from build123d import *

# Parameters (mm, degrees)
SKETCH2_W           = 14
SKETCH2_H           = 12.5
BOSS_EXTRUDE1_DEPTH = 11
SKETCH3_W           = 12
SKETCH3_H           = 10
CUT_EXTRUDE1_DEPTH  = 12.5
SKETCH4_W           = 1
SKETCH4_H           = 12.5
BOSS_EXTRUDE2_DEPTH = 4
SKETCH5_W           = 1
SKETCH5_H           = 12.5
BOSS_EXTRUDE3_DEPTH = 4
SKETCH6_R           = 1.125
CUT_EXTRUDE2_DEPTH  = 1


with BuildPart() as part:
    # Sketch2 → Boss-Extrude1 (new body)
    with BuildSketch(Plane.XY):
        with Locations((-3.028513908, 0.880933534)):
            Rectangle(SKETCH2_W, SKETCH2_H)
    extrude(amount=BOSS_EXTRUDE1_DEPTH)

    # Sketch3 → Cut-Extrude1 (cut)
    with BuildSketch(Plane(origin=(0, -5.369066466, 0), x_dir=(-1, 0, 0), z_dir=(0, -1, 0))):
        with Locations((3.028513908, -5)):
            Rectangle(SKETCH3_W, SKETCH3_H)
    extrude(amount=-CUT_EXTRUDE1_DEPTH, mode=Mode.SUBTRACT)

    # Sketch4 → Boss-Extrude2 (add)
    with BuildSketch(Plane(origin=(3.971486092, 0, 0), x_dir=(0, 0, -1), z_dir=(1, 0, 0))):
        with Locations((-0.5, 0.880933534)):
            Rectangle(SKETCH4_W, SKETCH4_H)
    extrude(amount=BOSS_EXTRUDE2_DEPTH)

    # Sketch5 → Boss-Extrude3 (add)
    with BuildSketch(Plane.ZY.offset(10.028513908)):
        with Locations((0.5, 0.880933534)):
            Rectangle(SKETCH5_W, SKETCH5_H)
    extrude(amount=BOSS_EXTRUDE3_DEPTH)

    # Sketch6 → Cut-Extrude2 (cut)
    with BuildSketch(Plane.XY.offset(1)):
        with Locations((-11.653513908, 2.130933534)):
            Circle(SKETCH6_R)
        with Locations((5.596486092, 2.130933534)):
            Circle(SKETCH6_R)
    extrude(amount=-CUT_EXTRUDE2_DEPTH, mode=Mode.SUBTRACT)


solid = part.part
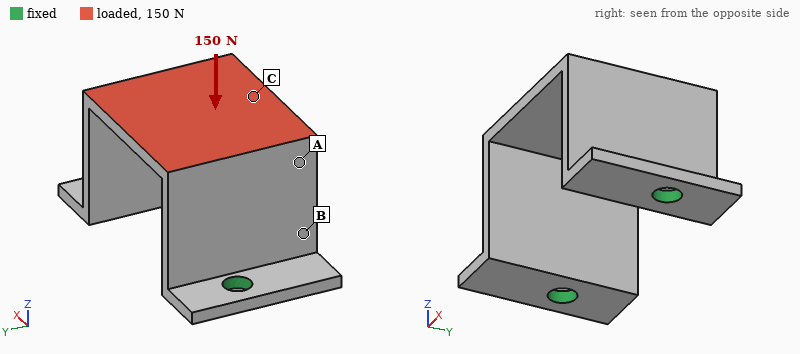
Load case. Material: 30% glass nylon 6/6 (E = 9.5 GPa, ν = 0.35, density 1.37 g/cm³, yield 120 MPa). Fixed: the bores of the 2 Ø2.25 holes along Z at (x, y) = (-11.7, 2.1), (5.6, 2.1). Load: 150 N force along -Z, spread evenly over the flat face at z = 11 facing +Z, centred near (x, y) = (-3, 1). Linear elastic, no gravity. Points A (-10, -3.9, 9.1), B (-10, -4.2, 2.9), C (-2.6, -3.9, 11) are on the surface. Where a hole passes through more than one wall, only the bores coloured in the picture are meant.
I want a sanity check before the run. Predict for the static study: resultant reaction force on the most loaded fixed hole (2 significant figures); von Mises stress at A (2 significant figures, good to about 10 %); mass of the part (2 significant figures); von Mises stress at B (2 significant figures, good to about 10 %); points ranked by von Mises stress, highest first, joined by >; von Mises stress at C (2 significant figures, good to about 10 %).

77 N
34 MPa
0.71 g
11 MPa
C > A > B
51 MPa
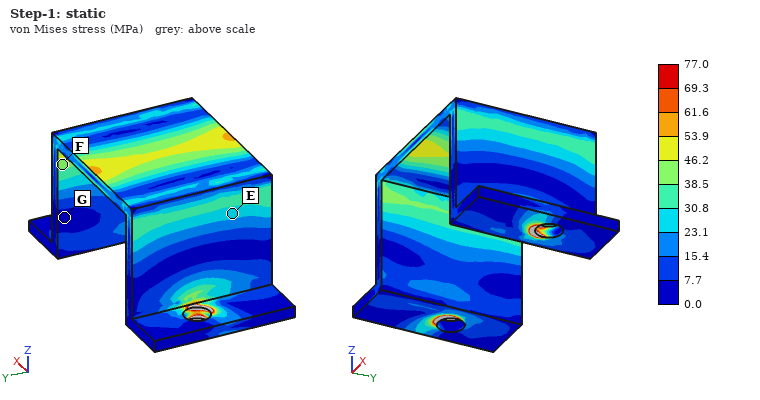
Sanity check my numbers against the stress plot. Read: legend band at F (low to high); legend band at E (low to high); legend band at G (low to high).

38.5 to 46.2 MPa
23.1 to 30.8 MPa
0.0 to 7.7 MPa
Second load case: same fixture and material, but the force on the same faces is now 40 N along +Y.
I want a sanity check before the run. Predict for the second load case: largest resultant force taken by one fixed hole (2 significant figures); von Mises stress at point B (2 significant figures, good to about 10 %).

20 N
13 MPa
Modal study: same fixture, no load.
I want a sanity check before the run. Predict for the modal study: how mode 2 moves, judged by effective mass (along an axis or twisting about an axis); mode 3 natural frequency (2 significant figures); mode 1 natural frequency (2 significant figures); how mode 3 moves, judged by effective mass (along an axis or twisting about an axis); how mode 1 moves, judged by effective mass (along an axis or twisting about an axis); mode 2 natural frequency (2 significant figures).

along Y
4800 Hz
3100 Hz
twisting about Z
along X
3500 Hz
